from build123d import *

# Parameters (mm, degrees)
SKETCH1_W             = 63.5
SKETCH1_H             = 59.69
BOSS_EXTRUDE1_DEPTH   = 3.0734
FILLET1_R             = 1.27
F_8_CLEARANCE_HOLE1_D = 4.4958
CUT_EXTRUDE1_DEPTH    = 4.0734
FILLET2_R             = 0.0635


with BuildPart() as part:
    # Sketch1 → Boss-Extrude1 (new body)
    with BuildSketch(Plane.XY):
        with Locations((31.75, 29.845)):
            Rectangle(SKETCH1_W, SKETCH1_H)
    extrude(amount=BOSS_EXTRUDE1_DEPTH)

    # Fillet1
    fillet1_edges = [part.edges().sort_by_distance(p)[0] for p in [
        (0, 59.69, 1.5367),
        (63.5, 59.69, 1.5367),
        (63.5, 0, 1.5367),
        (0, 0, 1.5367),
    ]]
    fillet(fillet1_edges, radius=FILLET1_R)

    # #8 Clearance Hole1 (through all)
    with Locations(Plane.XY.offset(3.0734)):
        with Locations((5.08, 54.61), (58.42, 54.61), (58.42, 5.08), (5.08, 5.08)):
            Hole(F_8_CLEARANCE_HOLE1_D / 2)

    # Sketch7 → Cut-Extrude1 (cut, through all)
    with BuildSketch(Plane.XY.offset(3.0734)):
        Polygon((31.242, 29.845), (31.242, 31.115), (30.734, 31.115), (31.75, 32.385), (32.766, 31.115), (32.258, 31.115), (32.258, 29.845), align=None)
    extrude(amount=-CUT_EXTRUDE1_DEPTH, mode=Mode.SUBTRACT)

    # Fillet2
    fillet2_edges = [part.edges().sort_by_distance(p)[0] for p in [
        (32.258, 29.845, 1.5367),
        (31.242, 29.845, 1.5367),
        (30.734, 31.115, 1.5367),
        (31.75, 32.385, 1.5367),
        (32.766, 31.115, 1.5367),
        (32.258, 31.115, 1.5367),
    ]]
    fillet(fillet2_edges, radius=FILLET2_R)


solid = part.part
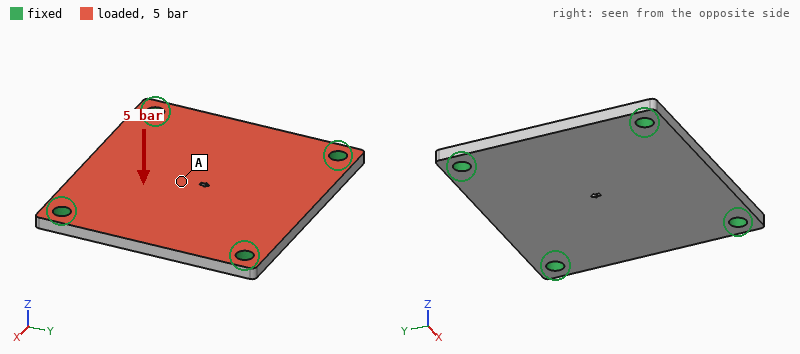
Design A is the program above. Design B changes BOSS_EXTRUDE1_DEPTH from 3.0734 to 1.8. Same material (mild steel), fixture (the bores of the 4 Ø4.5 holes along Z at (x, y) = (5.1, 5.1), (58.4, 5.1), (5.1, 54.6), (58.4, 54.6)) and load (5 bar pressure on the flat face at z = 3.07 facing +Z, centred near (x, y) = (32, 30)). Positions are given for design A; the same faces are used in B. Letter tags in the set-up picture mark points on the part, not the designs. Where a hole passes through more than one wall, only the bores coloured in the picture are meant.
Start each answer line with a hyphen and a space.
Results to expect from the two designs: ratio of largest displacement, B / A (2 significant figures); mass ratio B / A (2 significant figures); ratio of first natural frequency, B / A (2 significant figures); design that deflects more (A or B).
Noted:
- 4.7
- 0.59
- 0.61
- B
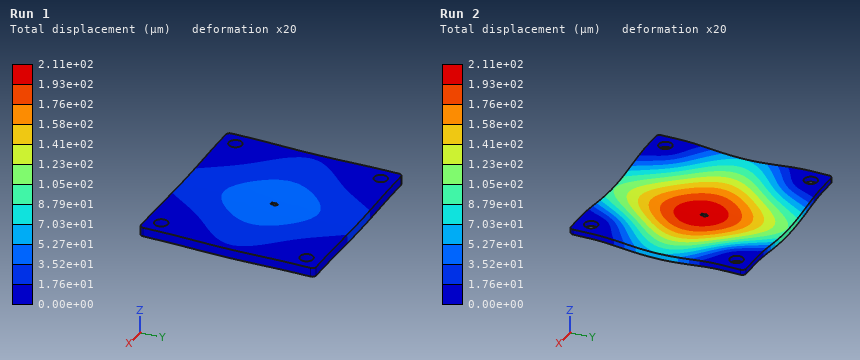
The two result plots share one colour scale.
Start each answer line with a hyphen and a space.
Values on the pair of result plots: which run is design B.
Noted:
- Run 2
